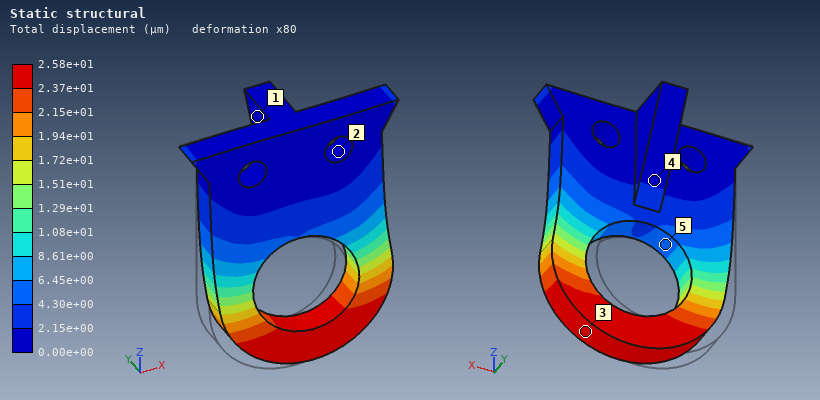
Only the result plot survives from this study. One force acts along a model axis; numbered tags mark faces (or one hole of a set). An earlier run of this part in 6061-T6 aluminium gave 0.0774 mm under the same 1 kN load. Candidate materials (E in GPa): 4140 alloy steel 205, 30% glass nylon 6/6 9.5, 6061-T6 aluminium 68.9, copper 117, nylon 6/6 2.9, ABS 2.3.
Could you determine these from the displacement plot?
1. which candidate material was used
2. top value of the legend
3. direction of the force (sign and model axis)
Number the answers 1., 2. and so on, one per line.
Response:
1. 4140 alloy steel
2. 2.58e+01 µm
3. +X
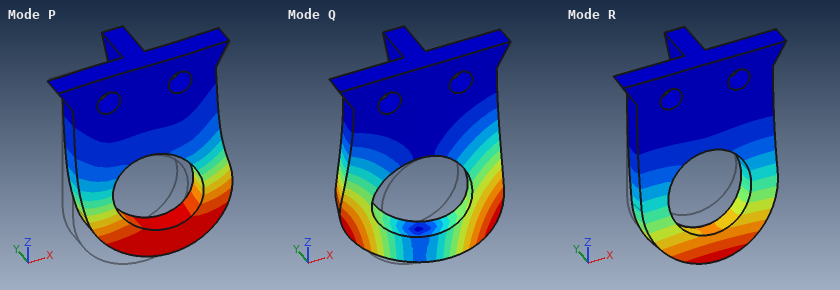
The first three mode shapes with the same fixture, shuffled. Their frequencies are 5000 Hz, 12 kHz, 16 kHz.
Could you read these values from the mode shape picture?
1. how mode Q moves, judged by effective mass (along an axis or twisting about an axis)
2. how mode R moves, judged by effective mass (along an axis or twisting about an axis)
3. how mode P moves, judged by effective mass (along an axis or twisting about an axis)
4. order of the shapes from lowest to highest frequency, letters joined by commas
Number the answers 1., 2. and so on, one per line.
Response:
1. twisting about Z
2. along Y
3. along X
4. R, Q, P
